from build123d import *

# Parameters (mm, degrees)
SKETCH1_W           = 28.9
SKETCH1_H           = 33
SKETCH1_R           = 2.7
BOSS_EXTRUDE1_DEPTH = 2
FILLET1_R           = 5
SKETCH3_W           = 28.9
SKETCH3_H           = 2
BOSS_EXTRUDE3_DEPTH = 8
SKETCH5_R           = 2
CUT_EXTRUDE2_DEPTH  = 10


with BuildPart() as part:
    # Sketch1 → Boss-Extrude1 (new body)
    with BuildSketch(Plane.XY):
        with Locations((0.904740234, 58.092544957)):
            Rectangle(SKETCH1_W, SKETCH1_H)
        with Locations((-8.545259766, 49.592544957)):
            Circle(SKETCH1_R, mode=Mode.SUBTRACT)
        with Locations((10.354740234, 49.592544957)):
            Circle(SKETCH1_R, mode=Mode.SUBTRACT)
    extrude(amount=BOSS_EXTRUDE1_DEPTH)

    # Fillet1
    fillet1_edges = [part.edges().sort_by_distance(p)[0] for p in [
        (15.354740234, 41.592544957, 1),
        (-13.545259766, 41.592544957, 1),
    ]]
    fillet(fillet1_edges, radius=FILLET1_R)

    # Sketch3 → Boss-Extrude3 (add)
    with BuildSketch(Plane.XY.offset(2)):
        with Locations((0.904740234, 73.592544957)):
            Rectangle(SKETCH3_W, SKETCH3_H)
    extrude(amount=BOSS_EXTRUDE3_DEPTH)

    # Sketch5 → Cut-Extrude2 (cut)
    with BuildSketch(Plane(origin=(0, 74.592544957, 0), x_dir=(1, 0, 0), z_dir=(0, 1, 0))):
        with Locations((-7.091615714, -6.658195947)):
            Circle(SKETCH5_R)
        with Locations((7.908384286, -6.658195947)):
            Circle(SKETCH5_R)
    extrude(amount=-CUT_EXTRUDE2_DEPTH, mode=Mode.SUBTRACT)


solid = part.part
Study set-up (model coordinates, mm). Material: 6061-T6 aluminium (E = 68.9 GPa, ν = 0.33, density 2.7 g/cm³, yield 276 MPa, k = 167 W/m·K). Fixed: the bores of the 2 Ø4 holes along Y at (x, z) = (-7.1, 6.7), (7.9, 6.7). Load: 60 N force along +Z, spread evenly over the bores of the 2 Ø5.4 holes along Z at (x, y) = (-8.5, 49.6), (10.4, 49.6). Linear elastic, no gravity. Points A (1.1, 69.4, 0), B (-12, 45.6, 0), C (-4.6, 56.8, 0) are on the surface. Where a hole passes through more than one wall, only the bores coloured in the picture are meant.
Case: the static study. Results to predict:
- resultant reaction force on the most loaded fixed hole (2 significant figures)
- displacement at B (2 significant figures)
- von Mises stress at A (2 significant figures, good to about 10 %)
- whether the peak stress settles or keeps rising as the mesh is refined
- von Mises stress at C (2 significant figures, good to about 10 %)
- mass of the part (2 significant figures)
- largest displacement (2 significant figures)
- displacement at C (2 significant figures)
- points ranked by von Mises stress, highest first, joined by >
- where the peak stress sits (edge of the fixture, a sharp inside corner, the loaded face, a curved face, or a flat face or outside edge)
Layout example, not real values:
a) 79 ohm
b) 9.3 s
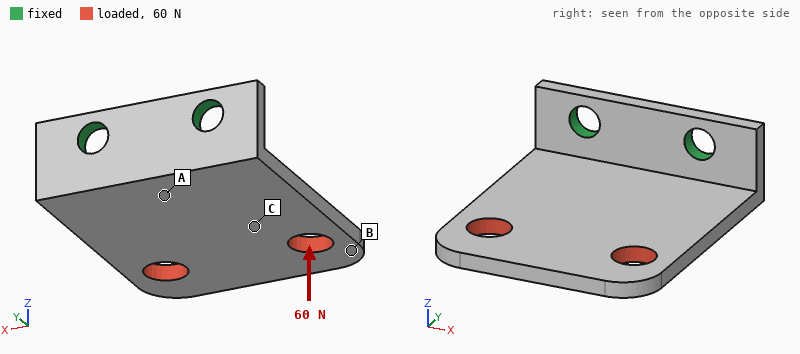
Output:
a) 34 N
b) 0.36 mm
c) 56 MPa
d) keeps rising
e) 21 MPa
f) 6.0 g
g) 0.43 mm
h) 0.18 mm
i) A > C > B
j) edge of the fixture
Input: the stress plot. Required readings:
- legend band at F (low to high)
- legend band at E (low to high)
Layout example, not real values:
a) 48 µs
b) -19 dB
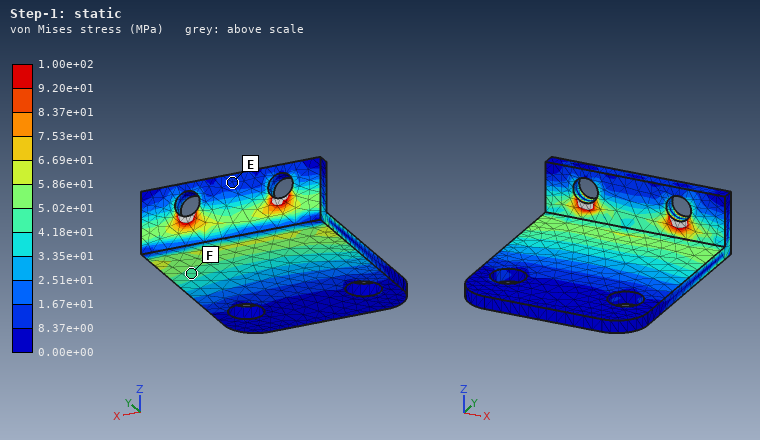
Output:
a) 4.18e+01 to 5.02e+01 MPa
b) 8.37e+00 to 1.67e+01 MPa
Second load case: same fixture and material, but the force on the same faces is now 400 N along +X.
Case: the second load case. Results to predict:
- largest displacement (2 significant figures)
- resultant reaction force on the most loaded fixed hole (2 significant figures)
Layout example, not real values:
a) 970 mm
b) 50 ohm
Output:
a) 0.14 mm
b) 600 N
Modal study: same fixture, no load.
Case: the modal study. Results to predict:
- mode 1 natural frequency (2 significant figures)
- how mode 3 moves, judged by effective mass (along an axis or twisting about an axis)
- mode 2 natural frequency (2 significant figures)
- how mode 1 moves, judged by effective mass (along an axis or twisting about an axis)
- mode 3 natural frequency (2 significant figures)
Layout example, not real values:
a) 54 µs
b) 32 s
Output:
a) 1400 Hz
b) along X
c) 4000 Hz
d) along Z
e) 6400 Hz
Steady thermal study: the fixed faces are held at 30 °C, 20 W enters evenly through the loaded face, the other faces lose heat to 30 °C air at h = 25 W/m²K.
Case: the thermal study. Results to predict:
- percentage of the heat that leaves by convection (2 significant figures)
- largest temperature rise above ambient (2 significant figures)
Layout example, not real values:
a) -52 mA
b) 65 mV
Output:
a) 9.3 %
b) 63 K
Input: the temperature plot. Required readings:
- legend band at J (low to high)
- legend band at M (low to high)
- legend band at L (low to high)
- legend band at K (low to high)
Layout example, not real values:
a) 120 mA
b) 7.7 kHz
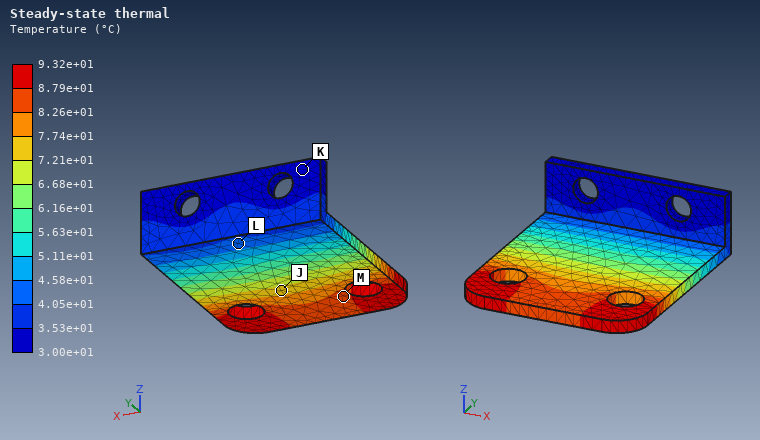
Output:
a) 7.21e+01 to 7.74e+01 °C
b) 8.26e+01 to 8.79e+01 °C
c) 4.05e+01 to 4.58e+01 °C
d) 3.00e+01 to 3.53e+01 °C
